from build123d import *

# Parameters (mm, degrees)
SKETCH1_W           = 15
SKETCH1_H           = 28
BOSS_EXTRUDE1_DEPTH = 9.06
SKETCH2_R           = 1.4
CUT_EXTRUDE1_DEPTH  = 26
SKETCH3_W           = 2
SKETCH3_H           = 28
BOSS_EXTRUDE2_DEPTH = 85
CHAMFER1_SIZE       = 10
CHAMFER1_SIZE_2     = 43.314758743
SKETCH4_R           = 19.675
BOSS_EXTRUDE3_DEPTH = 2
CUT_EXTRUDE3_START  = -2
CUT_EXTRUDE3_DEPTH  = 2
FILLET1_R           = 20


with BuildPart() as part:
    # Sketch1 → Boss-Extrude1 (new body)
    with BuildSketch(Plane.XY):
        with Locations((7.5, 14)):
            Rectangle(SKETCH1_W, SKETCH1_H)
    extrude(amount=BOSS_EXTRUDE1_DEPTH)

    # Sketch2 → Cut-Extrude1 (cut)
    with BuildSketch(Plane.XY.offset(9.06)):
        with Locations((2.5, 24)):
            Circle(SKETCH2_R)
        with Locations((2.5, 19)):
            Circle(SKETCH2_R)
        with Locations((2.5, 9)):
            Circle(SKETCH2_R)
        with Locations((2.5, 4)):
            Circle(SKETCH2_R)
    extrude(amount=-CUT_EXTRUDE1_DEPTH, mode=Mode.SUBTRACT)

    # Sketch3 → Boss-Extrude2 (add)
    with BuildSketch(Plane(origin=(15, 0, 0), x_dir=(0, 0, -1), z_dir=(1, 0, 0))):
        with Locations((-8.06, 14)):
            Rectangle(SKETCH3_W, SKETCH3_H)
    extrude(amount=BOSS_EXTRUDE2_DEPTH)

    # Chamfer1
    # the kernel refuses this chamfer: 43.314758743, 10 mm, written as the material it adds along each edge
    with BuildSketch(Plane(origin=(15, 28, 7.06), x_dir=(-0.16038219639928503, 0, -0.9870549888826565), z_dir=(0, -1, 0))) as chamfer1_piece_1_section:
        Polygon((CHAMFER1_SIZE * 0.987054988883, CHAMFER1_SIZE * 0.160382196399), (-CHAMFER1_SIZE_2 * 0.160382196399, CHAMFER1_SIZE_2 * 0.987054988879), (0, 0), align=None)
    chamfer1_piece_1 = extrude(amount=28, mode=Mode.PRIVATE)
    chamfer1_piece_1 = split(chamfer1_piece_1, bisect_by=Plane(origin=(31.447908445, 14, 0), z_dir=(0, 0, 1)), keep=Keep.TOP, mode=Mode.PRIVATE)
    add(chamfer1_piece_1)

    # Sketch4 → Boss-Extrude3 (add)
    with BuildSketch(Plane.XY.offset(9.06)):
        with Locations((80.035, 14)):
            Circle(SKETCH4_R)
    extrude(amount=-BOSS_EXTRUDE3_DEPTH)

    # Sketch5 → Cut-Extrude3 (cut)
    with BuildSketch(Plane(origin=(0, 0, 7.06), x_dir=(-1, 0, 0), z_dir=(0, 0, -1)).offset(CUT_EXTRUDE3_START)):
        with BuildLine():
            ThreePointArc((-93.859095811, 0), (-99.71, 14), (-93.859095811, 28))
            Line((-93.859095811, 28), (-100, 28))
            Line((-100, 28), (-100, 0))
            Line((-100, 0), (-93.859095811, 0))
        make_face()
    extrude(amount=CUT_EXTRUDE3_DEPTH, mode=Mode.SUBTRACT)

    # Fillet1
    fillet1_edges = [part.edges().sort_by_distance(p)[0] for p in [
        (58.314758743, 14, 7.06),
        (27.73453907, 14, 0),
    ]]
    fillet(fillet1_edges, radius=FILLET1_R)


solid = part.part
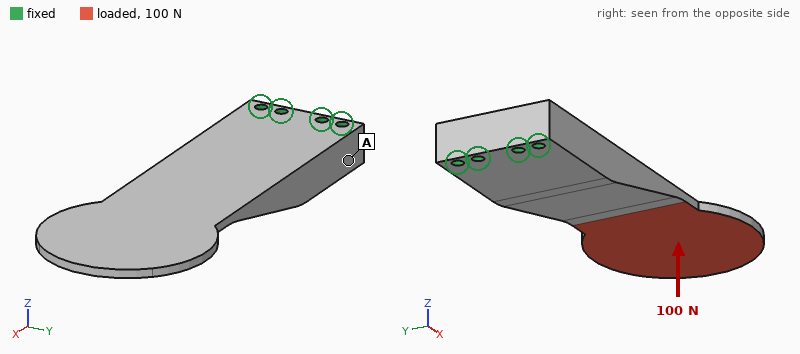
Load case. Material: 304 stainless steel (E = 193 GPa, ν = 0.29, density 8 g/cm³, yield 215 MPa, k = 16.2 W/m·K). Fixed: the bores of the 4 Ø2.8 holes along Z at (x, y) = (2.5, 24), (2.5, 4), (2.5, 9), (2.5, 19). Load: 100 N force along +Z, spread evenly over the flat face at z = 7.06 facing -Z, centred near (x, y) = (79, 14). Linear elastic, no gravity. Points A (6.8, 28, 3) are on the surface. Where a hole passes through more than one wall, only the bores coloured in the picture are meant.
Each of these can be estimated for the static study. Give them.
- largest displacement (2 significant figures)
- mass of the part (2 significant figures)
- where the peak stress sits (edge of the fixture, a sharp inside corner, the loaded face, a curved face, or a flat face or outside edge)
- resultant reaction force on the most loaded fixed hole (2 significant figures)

0.40 mm
110 g
a flat face or outside edge
60 N
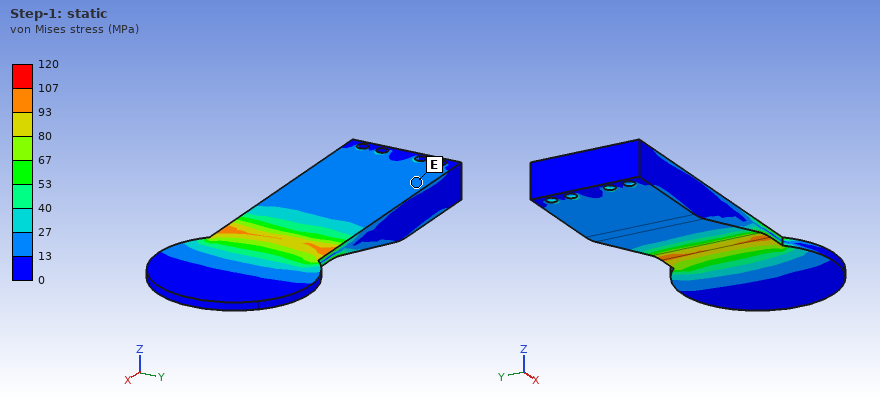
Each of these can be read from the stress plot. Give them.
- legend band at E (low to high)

13 to 27 MPa
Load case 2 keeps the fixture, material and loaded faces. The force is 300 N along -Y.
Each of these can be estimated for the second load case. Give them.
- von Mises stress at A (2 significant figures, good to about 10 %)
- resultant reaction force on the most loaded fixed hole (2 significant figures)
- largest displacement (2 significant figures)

14 MPa
920 N
38 µm
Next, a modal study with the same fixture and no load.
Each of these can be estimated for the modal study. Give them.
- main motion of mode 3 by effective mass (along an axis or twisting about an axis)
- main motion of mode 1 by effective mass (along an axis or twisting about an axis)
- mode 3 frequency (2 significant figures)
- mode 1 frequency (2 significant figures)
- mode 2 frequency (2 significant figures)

along Z
along Z
2700 Hz
710 Hz
2100 Hz
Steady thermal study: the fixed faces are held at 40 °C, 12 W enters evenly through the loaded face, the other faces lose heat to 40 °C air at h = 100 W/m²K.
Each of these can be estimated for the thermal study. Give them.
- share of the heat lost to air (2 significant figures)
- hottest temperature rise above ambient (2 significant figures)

96 %
72 K
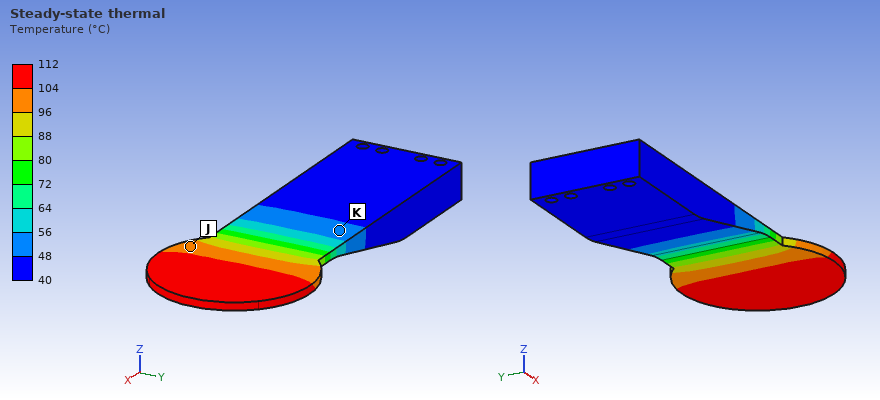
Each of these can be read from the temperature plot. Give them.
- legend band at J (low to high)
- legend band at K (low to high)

96 to 104 °C
48 to 56 °C
